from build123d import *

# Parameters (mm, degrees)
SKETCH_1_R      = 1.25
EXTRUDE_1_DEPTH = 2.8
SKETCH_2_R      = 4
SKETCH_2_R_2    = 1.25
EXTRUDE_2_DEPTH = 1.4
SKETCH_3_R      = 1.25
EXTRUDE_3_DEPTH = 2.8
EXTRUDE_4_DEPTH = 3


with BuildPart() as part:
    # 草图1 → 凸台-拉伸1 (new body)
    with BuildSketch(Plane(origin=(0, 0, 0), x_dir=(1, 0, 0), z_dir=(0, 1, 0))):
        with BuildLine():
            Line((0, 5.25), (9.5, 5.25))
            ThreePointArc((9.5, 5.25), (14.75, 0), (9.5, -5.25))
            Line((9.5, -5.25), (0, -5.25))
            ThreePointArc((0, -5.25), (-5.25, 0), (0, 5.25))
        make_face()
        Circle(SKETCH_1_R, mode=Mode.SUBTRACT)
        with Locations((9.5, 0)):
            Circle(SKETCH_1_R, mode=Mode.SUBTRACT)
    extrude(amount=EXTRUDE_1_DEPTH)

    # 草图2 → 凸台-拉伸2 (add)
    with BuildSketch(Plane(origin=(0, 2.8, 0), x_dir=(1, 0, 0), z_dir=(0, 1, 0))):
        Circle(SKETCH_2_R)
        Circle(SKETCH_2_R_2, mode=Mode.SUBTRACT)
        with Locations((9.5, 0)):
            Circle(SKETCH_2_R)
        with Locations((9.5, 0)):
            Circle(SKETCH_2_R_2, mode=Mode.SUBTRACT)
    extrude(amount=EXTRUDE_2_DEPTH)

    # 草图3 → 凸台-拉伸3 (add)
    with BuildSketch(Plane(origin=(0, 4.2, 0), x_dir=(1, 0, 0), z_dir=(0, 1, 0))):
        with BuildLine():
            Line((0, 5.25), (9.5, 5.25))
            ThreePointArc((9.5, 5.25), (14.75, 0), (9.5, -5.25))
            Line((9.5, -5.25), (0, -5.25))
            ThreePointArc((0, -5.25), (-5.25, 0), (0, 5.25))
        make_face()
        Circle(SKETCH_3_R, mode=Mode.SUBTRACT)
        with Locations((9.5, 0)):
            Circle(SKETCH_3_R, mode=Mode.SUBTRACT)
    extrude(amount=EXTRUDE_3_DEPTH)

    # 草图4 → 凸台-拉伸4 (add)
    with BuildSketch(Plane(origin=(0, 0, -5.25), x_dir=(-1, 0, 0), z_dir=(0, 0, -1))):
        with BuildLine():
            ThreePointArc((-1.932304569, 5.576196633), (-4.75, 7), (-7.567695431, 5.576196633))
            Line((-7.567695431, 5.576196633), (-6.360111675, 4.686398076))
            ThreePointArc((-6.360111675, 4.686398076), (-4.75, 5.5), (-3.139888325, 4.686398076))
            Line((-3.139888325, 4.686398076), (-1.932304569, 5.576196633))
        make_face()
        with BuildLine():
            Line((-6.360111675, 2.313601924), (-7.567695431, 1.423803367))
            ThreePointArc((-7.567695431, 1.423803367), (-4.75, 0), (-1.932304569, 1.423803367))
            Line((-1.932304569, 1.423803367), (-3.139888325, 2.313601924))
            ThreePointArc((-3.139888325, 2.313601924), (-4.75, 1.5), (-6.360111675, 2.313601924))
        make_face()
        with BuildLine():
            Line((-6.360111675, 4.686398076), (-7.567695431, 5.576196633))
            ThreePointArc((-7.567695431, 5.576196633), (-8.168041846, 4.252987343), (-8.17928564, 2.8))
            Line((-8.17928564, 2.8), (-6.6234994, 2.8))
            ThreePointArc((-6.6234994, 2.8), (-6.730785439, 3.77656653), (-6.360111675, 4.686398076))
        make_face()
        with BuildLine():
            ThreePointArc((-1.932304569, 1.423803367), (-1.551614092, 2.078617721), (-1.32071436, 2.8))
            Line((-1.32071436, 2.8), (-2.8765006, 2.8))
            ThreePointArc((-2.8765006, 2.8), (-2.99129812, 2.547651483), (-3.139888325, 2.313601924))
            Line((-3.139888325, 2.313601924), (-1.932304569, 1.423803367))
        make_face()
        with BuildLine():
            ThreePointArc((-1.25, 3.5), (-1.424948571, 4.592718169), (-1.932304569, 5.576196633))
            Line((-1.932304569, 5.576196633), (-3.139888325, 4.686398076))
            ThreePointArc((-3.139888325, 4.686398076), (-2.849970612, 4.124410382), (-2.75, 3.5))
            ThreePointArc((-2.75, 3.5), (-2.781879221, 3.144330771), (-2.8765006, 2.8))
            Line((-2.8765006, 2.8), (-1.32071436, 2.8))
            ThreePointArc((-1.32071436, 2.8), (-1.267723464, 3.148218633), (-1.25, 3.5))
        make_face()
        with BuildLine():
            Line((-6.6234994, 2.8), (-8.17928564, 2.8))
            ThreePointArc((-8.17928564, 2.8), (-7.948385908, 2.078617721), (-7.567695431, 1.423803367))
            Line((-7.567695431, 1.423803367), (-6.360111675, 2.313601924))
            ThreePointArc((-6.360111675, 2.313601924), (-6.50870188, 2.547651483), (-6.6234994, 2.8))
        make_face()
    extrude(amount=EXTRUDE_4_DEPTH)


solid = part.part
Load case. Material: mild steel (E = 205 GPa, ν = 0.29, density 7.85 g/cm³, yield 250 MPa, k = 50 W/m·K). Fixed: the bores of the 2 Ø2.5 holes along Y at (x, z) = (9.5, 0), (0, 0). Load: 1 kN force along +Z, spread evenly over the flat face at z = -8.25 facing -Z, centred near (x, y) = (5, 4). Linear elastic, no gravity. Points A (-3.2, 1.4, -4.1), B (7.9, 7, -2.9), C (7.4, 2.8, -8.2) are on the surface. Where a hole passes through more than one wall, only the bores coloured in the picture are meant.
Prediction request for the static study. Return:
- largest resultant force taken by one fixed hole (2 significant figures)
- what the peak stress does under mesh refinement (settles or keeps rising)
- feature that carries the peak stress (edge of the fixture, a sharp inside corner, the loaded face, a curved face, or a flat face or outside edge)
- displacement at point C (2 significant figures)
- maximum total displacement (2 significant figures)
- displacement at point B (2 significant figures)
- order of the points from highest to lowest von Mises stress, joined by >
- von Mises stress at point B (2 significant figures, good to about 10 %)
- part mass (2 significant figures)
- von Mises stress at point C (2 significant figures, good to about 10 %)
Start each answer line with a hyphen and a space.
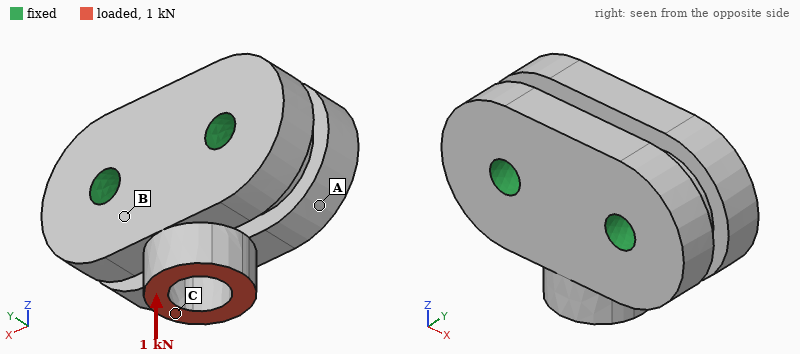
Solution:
- 530 N
- keeps rising
- a sharp inside corner
- 1.3 µm
- 1.3 µm
- 0.28 µm
- C > B > A
- 21 MPa
- 9.4 g
- 38 MPa
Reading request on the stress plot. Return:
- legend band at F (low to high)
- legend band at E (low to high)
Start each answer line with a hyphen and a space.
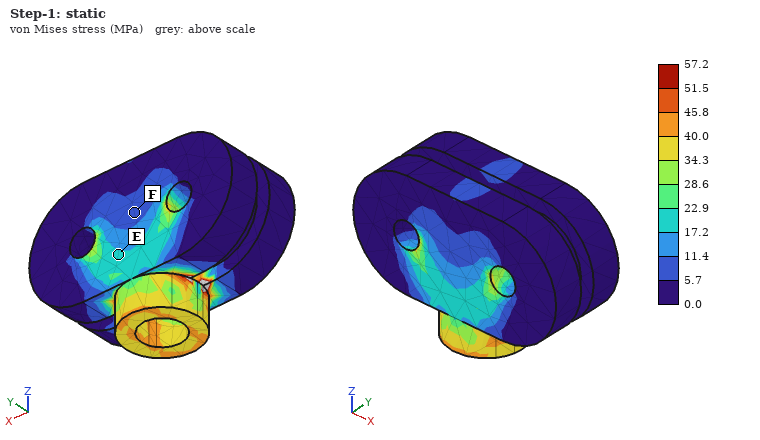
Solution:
- 5.7 to 11.4 MPa
- 17.2 to 22.9 MPa
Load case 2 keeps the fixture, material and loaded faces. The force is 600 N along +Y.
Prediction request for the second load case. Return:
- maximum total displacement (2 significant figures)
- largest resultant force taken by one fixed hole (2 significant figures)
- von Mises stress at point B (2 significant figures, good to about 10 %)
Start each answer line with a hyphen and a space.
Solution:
- 6.5 µm
- 300 N
- 59 MPa
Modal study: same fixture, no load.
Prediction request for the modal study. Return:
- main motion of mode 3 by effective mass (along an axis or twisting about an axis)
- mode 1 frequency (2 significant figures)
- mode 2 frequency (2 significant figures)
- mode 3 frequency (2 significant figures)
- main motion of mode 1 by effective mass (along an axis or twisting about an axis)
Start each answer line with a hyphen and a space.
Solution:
- along Y
- 75 kHz
- 110 kHz
- 110 kHz
- along Y
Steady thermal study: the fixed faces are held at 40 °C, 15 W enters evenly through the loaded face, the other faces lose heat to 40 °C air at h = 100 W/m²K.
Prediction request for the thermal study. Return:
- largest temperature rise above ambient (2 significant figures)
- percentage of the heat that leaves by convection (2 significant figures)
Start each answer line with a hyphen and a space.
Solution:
- 62 K
- 5.6 %
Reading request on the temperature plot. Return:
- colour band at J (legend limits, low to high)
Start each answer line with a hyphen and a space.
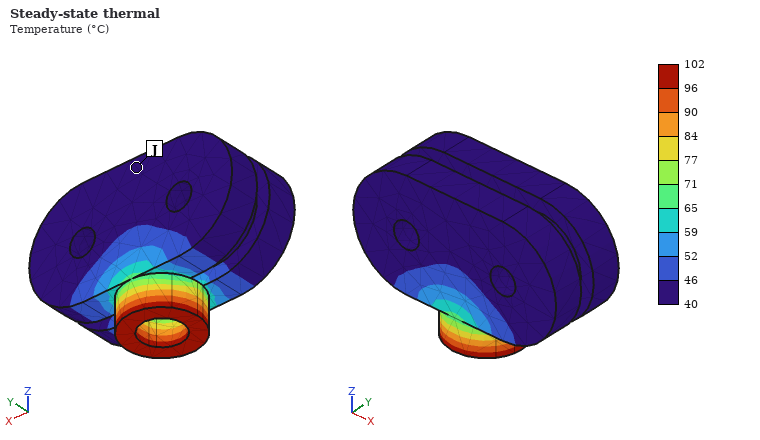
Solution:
- 40 to 46 °C
